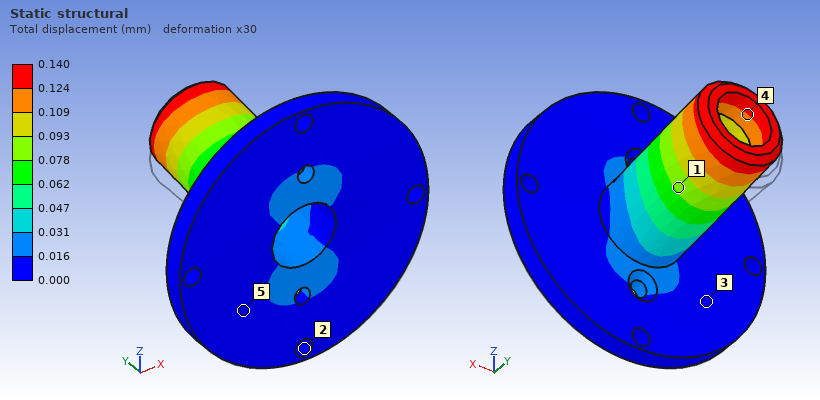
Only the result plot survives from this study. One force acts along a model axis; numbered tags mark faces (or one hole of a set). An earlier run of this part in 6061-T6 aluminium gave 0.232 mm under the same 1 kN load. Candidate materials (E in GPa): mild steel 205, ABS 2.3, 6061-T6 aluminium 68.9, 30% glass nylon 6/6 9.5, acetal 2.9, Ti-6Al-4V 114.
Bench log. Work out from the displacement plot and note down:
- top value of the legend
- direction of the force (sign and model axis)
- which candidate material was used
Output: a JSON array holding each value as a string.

["0.140 mm", "+Z", "Ti-6Al-4V"]
